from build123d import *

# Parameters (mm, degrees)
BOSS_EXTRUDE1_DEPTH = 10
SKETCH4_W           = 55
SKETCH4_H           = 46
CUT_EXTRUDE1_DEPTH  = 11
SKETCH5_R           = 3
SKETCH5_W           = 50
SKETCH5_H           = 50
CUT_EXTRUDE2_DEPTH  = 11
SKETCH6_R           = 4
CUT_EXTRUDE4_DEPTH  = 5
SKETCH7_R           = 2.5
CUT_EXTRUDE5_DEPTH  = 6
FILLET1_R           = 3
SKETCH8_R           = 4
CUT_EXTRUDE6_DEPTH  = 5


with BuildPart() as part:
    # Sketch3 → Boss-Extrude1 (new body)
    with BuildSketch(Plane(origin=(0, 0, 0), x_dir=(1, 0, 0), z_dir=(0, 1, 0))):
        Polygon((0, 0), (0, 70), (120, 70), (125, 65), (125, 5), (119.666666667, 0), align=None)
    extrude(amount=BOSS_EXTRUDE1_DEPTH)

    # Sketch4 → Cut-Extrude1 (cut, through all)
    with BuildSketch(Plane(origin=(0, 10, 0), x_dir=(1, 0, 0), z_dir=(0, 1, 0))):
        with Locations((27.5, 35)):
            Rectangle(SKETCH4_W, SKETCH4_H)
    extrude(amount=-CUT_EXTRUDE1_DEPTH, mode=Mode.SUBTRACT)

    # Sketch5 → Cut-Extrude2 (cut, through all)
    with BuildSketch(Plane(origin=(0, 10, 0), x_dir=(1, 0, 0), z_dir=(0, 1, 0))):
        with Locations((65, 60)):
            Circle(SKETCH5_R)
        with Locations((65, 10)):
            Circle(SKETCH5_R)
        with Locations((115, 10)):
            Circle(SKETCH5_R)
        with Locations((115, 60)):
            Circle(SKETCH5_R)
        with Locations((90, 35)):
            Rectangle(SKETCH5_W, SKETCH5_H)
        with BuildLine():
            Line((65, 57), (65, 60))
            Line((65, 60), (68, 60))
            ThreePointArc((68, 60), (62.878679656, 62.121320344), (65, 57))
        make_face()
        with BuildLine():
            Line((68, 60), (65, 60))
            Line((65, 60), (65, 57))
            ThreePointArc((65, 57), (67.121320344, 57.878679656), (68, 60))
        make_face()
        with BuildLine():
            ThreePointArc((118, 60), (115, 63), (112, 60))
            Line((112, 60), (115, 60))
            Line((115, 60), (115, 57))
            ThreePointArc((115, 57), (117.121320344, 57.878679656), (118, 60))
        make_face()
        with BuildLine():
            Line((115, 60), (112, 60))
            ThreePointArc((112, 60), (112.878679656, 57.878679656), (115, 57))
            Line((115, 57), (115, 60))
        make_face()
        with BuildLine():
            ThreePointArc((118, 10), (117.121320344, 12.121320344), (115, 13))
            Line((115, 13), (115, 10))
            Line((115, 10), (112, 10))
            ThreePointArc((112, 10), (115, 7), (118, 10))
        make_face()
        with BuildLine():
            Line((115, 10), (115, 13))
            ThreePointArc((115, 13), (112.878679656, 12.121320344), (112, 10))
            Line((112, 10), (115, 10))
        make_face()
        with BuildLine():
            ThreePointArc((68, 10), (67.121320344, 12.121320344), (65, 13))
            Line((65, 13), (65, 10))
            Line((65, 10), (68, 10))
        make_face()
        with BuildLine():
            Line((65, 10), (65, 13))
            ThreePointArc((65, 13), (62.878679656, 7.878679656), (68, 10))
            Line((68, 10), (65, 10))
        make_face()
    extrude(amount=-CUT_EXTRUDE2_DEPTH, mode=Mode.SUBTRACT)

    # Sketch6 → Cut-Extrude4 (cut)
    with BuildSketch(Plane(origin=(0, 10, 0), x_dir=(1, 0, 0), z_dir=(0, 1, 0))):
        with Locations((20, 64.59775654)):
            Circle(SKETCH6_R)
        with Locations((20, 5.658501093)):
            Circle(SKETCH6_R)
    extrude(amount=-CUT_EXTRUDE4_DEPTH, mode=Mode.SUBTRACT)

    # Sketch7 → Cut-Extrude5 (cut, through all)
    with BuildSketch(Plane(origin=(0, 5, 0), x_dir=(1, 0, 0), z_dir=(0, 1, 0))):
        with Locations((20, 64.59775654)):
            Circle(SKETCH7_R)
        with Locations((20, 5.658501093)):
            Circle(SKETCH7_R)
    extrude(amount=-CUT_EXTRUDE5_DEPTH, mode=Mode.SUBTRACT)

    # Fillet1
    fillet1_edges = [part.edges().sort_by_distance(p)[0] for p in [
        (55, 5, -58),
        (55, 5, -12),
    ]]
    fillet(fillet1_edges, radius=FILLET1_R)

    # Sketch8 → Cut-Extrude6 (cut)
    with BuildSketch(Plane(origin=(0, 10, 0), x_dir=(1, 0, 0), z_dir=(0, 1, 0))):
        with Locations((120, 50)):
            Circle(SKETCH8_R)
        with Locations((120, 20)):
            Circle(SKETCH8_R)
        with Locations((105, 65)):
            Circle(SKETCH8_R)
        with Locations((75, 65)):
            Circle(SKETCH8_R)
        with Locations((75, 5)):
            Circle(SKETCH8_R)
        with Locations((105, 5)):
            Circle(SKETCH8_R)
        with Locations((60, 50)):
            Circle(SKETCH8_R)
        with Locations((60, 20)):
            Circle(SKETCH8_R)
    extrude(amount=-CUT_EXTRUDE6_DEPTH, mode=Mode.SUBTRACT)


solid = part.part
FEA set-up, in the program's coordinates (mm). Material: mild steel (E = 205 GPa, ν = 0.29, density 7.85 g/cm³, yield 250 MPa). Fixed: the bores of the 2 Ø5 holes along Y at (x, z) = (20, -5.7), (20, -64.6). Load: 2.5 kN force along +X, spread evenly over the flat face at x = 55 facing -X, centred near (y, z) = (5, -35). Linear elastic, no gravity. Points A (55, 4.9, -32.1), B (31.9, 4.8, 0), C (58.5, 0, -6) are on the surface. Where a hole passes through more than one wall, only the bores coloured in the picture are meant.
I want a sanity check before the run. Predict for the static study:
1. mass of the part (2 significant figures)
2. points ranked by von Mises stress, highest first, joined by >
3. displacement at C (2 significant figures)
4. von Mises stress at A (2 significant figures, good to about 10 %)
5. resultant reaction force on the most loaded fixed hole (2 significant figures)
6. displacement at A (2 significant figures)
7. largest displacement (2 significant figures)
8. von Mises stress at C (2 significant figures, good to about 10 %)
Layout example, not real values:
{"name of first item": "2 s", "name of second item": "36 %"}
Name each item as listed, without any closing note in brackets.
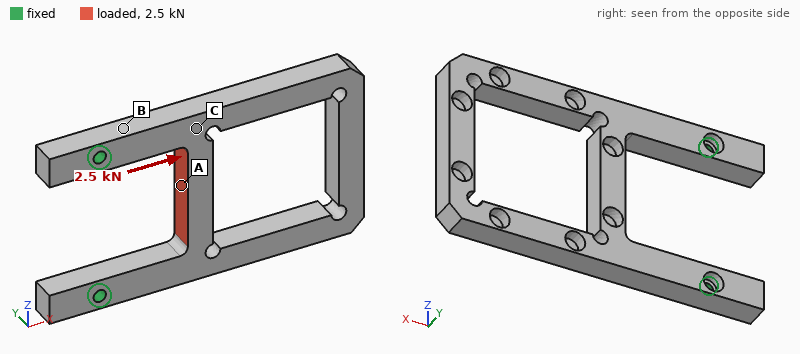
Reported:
{"mass of the part": "260 g", "points ranked by von Mises stress, highest first, joined by >": "A > C > B", "displacement at C": "7.6 µm", "von Mises stress at A": "53 MPa", "resultant reaction force on the most loaded fixed hole": "1.3 kN", "displacement at A": "22 µm", "largest displacement": "28 µm", "von Mises stress at C": "23 MPa"}
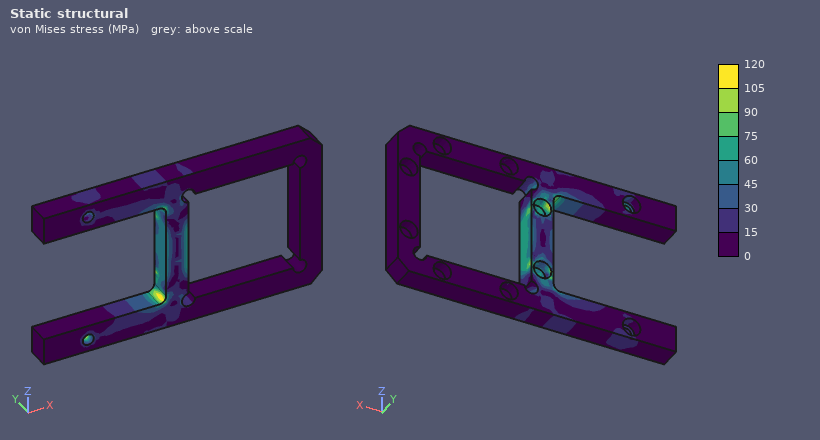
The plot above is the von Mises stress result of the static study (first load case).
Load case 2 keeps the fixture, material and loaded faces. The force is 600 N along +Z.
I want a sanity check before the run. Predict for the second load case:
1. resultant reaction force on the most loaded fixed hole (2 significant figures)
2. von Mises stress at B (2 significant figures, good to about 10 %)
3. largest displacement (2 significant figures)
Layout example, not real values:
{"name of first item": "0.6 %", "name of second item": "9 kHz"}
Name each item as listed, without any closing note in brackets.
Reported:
{"resultant reaction force on the most loaded fixed hole": "330 N", "von Mises stress at B": "15 MPa", "largest displacement": "29 µm"}
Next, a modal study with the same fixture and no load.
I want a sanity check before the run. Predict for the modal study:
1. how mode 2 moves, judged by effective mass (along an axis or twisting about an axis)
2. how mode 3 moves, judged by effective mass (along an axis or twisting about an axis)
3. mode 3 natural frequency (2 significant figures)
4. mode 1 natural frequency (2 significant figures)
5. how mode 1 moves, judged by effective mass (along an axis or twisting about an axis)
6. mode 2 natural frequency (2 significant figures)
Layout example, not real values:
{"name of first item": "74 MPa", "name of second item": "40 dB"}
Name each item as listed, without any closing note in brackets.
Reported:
{"how mode 2 moves, judged by effective mass": "along Z", "how mode 3 moves, judged by effective mass": "twisting about X", "mode 3 natural frequency": "1300 Hz", "mode 1 natural frequency": "520 Hz", "how mode 1 moves, judged by effective mass": "along Y", "mode 2 natural frequency": "1100 Hz"}
